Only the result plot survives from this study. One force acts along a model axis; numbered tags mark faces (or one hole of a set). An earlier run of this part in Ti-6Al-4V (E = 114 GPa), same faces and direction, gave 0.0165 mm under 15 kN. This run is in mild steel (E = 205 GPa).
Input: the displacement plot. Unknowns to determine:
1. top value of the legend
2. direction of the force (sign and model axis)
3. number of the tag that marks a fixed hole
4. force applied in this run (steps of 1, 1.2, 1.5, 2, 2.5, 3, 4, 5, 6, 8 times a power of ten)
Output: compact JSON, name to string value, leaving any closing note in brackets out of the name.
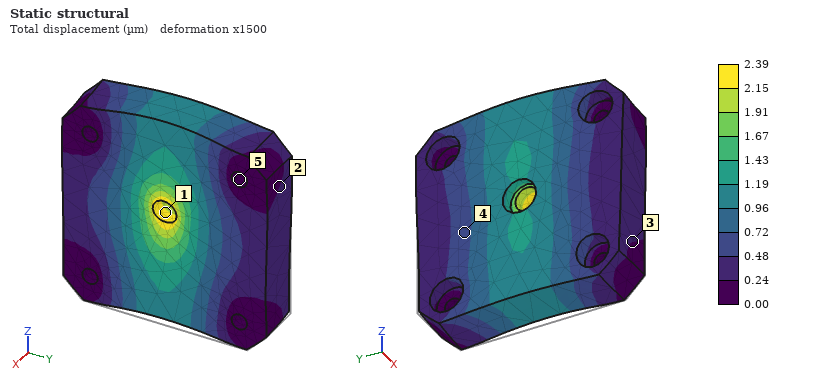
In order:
{"top value of the legend": "2.39 µm", "direction of the force": "+Z", "number of the tag that marks a fixed hole": "5", "force applied in this run": "4 kN"}
